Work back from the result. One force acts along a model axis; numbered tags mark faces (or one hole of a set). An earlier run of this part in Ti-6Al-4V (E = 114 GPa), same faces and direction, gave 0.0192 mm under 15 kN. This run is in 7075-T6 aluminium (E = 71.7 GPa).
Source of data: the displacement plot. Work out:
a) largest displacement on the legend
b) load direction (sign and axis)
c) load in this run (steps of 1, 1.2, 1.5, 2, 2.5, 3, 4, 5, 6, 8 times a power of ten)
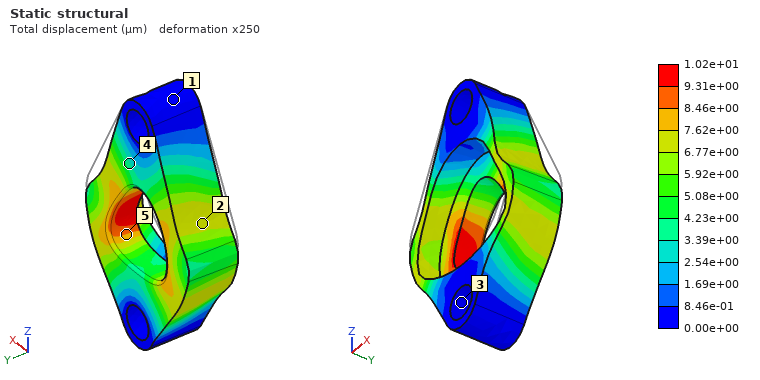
1.02e+01 µm
-Z
5 kN
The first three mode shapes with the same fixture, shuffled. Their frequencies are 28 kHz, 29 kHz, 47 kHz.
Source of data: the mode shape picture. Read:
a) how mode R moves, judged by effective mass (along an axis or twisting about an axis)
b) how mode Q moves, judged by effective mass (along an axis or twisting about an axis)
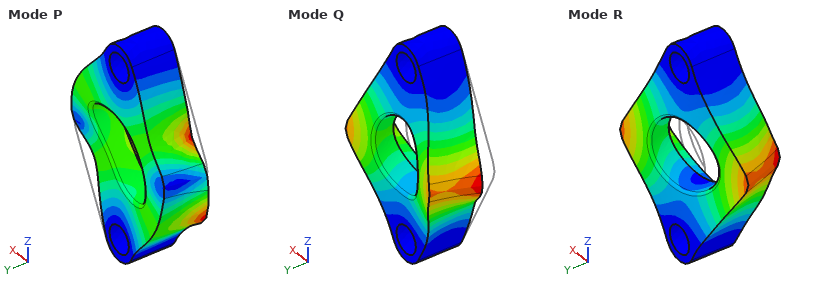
twisting about Z
along Y
